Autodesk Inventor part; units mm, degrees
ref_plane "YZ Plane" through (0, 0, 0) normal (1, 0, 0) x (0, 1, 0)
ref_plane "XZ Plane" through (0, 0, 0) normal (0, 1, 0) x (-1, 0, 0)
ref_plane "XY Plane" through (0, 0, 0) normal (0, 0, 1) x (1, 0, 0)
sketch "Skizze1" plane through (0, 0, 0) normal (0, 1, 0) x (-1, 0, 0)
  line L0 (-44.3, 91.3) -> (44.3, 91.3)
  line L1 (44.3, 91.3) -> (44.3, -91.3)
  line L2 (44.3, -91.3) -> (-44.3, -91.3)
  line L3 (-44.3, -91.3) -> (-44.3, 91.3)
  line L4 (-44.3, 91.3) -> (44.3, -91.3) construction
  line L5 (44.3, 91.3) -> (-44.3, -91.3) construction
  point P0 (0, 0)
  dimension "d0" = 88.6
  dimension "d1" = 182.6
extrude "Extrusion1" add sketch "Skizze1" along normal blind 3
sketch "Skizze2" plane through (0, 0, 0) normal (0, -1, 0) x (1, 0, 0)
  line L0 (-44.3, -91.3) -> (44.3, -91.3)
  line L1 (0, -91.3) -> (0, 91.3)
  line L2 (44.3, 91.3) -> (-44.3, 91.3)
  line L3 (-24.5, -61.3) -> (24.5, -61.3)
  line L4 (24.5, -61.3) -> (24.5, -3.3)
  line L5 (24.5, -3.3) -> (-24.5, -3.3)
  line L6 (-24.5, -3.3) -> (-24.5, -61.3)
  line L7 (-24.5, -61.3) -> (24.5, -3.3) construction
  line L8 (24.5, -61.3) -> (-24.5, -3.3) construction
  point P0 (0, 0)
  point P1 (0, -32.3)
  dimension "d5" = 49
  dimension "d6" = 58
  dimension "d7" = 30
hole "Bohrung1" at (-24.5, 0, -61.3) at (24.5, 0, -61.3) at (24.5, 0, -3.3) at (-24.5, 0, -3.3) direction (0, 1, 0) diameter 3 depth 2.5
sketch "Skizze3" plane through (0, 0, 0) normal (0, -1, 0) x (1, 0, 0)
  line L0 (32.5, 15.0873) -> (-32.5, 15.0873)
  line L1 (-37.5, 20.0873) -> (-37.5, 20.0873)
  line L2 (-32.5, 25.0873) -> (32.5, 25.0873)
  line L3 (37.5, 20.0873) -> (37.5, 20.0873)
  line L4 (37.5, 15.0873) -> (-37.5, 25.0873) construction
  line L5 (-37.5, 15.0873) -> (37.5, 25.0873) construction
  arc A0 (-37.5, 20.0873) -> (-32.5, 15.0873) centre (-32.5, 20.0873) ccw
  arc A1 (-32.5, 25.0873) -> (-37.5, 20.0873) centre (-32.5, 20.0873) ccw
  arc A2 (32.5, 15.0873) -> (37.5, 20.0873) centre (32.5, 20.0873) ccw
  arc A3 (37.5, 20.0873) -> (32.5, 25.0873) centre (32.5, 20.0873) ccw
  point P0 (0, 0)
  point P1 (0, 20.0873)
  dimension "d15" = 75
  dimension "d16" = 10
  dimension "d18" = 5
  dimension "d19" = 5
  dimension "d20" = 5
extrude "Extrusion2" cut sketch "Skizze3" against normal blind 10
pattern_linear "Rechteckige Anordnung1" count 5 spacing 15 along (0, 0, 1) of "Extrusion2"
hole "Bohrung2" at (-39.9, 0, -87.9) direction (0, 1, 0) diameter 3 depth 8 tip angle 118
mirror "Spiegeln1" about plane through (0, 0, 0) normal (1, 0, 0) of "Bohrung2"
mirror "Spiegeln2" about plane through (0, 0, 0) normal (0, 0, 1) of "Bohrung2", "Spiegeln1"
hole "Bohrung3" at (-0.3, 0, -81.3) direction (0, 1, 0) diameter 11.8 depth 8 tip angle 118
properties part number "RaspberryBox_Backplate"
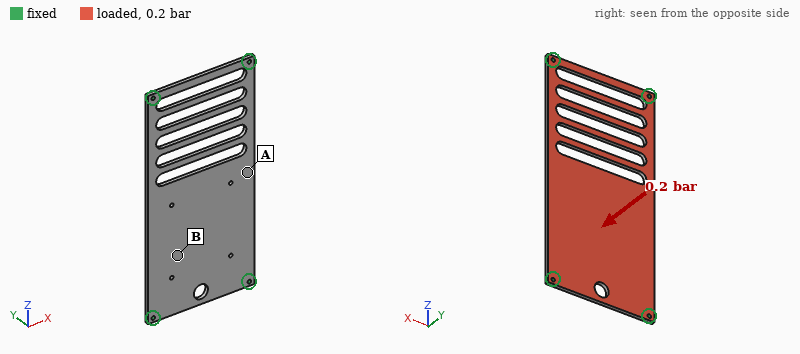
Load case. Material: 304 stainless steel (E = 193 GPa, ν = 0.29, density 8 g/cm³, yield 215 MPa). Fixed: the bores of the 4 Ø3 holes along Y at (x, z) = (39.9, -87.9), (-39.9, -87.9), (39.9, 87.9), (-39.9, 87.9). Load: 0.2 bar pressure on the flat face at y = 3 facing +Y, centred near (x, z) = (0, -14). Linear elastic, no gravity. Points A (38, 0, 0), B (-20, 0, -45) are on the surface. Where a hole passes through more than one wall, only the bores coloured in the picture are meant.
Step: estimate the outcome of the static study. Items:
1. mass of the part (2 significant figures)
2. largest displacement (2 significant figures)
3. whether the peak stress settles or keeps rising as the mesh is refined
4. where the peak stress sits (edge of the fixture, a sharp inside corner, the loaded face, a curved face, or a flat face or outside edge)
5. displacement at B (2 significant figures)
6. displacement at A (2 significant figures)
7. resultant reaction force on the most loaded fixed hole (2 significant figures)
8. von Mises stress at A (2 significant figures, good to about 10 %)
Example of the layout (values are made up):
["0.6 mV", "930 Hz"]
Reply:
["300 g", "0.31 mm", "keeps rising", "edge of the fixture", "0.14 mm", "0.27 mm", "77 N", "24 MPa"]
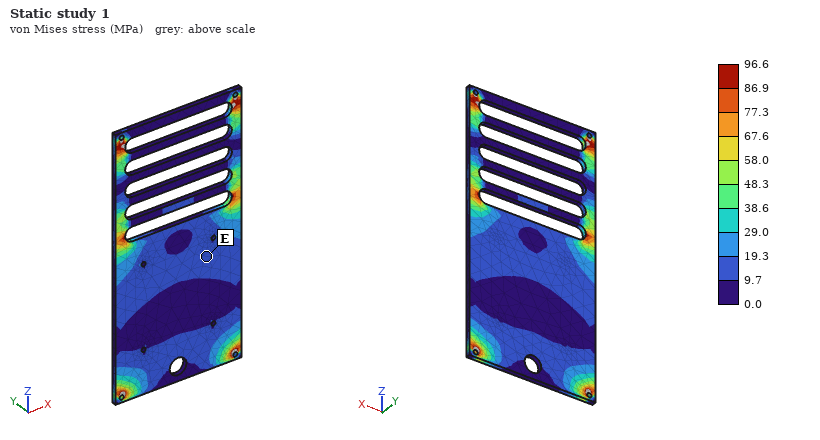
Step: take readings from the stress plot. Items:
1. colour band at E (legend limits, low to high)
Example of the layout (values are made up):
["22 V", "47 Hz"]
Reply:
["9.7 to 19.3 MPa"]
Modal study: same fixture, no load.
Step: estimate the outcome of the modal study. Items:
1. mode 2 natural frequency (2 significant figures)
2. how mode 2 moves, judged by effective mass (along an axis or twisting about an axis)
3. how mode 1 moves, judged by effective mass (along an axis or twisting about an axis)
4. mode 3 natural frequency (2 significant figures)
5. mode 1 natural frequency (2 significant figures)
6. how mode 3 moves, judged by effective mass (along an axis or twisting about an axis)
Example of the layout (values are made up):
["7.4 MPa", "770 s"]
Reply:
["690 Hz", "twisting about Z", "along Y", "960 Hz", "310 Hz", "twisting about X"]
